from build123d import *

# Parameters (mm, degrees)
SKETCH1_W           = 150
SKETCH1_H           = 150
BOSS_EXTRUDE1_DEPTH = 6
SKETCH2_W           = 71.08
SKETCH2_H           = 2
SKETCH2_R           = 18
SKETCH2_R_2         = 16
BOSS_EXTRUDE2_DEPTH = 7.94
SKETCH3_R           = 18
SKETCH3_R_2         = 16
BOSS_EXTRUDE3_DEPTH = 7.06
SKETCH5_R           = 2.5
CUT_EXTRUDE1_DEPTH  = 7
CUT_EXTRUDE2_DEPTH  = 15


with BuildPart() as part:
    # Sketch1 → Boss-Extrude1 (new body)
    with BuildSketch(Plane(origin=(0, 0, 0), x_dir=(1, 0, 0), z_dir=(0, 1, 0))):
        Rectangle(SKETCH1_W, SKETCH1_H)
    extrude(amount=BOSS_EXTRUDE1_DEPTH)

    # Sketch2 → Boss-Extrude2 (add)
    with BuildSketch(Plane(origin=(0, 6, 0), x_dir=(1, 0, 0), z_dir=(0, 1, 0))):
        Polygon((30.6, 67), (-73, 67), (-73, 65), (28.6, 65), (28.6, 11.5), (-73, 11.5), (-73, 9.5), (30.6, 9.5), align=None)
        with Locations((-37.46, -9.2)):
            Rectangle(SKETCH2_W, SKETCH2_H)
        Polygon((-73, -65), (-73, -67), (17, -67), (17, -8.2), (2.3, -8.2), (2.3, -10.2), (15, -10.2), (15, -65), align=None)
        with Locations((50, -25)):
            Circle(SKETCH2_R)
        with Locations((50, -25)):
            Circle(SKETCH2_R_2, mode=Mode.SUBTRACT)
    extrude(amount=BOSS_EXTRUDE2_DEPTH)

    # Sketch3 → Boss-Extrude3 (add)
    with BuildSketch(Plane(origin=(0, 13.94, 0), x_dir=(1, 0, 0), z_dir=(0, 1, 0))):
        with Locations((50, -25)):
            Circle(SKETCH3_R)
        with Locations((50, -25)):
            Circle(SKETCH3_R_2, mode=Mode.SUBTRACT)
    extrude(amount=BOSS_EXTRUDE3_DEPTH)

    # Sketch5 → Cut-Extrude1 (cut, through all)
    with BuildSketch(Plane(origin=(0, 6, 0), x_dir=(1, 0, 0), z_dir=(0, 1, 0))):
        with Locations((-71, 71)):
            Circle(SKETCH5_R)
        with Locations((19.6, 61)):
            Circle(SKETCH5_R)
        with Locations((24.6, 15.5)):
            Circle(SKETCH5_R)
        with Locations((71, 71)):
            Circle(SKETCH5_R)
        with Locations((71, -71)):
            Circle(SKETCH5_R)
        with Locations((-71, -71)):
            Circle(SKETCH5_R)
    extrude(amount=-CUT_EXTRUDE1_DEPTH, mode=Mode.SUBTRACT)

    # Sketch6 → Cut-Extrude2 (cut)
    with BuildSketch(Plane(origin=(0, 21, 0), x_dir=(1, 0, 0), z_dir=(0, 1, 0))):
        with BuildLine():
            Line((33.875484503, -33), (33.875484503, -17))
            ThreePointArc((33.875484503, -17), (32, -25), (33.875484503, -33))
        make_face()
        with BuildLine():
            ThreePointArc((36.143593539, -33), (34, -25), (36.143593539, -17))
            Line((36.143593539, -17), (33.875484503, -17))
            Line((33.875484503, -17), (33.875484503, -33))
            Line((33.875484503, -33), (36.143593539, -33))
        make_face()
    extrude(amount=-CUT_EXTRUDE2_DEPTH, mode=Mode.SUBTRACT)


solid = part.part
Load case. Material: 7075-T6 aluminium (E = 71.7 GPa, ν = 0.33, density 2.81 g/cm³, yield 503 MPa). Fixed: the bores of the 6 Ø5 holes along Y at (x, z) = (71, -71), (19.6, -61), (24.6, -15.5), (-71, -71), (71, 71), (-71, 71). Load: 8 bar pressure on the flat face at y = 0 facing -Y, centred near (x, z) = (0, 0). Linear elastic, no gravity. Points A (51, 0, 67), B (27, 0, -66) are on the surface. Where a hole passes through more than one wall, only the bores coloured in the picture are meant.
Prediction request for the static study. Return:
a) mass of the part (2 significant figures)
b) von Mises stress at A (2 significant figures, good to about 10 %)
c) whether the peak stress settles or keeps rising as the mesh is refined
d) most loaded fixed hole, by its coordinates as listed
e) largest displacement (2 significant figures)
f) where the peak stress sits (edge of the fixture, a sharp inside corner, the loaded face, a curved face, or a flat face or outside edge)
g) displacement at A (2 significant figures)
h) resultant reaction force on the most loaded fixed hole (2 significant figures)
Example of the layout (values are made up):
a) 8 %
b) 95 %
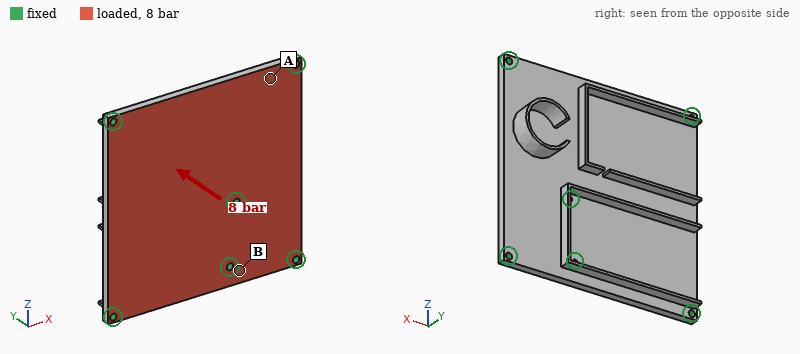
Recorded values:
a) 410 g
b) 69 MPa
c) keeps rising
d) (24.6, -15.5)
e) 0.84 mm
f) edge of the fixture
g) 0.19 mm
h) 7.5 kN
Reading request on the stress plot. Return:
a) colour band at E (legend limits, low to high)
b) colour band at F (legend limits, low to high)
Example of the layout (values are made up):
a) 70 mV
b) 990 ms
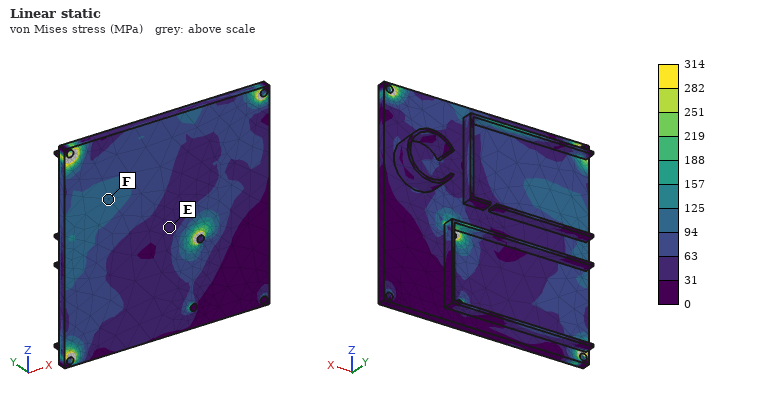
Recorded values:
a) 31 to 63 MPa
b) 94 to 125 MPa
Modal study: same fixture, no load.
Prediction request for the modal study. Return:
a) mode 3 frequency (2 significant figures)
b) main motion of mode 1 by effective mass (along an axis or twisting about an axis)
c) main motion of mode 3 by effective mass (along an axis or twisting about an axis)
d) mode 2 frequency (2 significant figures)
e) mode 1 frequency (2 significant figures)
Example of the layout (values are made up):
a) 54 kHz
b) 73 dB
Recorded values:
a) 2400 Hz
b) along Y
c) along Y
d) 1800 Hz
e) 1400 Hz
